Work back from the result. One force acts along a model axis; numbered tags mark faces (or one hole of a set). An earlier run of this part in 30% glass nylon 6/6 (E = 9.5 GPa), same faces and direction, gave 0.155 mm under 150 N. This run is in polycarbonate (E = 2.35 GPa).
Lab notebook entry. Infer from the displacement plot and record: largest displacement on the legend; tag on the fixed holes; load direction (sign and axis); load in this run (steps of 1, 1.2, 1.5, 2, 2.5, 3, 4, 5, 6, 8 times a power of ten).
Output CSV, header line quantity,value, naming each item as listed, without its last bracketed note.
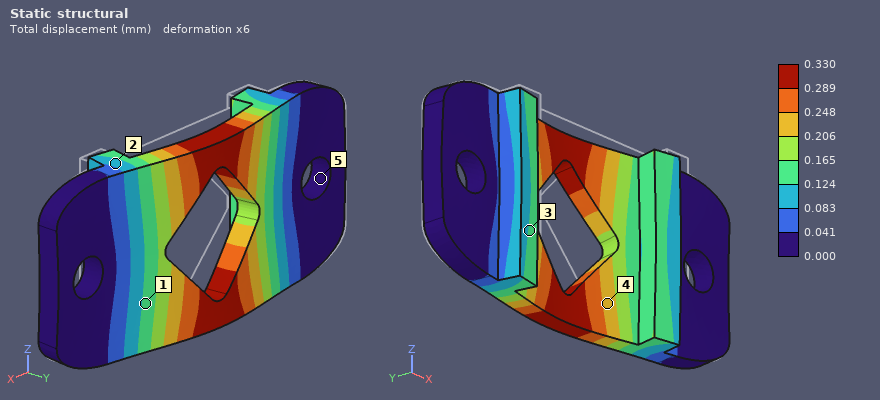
quantity,value
largest displacement on the legend,0.330 mm
tag on the fixed holes,5
load direction,+Y
load in this run,80 N
